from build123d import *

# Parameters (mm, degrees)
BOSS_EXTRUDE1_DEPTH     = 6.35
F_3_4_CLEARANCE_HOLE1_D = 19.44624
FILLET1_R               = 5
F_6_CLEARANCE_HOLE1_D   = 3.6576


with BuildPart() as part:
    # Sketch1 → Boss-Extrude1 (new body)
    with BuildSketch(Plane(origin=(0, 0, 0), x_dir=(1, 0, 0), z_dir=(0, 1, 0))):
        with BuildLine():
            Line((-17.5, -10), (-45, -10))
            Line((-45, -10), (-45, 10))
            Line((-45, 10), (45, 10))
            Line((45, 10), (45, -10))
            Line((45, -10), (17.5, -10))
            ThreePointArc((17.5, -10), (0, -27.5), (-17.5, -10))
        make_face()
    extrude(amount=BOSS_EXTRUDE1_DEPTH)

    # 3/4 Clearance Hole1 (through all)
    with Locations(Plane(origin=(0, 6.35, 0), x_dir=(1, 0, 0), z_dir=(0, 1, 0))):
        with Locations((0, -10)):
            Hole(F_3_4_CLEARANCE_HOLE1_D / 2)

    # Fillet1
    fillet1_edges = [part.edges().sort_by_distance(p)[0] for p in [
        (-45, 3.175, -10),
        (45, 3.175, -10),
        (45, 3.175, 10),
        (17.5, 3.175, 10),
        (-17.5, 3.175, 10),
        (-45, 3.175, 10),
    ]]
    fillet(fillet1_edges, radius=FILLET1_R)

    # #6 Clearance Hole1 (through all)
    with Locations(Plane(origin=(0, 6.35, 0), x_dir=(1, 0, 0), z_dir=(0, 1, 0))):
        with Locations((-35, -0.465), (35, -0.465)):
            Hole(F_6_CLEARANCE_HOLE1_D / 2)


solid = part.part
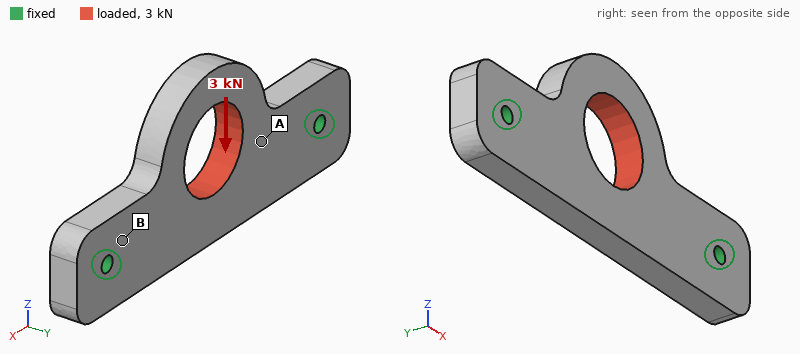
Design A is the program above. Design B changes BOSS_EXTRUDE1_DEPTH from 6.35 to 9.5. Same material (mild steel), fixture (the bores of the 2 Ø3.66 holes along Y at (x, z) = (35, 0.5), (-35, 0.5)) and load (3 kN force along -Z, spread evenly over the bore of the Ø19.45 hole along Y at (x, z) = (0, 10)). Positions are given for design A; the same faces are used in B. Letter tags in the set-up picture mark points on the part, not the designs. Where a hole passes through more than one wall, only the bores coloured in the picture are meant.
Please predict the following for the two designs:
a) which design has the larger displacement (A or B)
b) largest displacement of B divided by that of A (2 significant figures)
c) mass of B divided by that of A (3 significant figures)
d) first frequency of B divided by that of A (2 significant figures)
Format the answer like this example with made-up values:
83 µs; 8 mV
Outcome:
A; 0.67; 1.50; 1.4
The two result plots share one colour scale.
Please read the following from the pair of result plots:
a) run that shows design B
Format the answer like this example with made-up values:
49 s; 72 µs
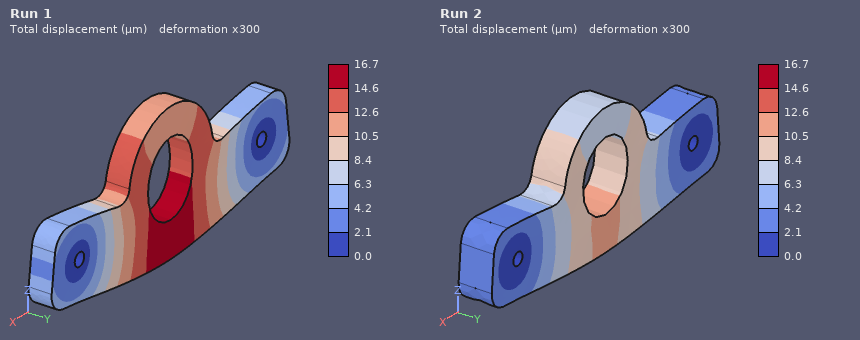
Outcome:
Run 2
